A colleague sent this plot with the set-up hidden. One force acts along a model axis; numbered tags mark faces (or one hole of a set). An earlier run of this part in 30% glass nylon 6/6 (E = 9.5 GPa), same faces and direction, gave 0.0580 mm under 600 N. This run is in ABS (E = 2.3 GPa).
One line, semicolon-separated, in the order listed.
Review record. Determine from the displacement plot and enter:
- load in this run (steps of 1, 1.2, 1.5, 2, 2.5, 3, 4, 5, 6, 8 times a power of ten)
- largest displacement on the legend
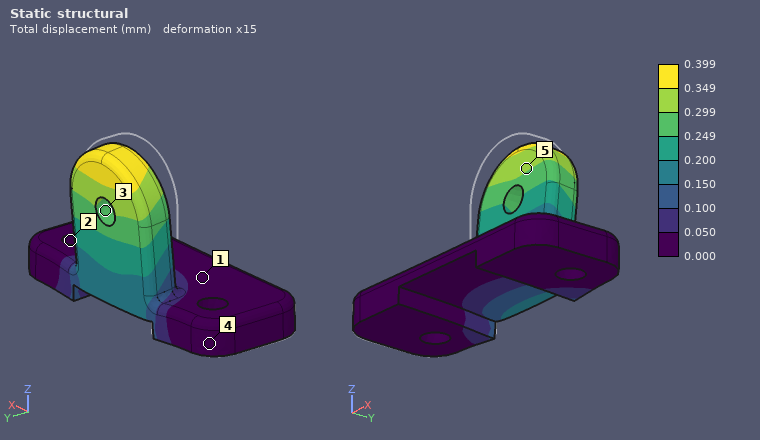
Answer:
1 kN; 0.399 mm
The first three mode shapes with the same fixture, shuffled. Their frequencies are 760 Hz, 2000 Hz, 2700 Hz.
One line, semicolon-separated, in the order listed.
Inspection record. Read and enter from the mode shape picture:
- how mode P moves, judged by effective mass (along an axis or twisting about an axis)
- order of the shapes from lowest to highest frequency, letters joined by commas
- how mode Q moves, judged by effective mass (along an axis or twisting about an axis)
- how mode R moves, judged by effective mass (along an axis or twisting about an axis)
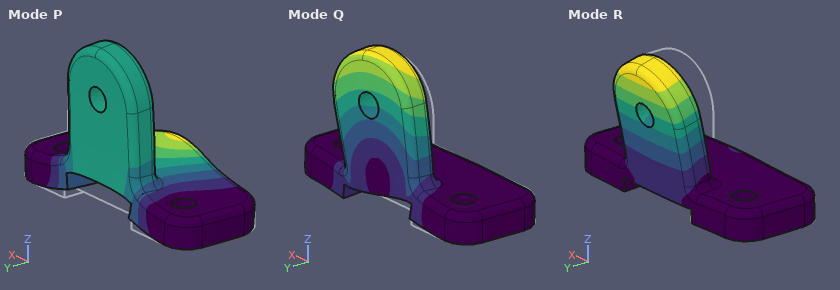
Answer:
along Z; R, Q, P; along X; along Y
